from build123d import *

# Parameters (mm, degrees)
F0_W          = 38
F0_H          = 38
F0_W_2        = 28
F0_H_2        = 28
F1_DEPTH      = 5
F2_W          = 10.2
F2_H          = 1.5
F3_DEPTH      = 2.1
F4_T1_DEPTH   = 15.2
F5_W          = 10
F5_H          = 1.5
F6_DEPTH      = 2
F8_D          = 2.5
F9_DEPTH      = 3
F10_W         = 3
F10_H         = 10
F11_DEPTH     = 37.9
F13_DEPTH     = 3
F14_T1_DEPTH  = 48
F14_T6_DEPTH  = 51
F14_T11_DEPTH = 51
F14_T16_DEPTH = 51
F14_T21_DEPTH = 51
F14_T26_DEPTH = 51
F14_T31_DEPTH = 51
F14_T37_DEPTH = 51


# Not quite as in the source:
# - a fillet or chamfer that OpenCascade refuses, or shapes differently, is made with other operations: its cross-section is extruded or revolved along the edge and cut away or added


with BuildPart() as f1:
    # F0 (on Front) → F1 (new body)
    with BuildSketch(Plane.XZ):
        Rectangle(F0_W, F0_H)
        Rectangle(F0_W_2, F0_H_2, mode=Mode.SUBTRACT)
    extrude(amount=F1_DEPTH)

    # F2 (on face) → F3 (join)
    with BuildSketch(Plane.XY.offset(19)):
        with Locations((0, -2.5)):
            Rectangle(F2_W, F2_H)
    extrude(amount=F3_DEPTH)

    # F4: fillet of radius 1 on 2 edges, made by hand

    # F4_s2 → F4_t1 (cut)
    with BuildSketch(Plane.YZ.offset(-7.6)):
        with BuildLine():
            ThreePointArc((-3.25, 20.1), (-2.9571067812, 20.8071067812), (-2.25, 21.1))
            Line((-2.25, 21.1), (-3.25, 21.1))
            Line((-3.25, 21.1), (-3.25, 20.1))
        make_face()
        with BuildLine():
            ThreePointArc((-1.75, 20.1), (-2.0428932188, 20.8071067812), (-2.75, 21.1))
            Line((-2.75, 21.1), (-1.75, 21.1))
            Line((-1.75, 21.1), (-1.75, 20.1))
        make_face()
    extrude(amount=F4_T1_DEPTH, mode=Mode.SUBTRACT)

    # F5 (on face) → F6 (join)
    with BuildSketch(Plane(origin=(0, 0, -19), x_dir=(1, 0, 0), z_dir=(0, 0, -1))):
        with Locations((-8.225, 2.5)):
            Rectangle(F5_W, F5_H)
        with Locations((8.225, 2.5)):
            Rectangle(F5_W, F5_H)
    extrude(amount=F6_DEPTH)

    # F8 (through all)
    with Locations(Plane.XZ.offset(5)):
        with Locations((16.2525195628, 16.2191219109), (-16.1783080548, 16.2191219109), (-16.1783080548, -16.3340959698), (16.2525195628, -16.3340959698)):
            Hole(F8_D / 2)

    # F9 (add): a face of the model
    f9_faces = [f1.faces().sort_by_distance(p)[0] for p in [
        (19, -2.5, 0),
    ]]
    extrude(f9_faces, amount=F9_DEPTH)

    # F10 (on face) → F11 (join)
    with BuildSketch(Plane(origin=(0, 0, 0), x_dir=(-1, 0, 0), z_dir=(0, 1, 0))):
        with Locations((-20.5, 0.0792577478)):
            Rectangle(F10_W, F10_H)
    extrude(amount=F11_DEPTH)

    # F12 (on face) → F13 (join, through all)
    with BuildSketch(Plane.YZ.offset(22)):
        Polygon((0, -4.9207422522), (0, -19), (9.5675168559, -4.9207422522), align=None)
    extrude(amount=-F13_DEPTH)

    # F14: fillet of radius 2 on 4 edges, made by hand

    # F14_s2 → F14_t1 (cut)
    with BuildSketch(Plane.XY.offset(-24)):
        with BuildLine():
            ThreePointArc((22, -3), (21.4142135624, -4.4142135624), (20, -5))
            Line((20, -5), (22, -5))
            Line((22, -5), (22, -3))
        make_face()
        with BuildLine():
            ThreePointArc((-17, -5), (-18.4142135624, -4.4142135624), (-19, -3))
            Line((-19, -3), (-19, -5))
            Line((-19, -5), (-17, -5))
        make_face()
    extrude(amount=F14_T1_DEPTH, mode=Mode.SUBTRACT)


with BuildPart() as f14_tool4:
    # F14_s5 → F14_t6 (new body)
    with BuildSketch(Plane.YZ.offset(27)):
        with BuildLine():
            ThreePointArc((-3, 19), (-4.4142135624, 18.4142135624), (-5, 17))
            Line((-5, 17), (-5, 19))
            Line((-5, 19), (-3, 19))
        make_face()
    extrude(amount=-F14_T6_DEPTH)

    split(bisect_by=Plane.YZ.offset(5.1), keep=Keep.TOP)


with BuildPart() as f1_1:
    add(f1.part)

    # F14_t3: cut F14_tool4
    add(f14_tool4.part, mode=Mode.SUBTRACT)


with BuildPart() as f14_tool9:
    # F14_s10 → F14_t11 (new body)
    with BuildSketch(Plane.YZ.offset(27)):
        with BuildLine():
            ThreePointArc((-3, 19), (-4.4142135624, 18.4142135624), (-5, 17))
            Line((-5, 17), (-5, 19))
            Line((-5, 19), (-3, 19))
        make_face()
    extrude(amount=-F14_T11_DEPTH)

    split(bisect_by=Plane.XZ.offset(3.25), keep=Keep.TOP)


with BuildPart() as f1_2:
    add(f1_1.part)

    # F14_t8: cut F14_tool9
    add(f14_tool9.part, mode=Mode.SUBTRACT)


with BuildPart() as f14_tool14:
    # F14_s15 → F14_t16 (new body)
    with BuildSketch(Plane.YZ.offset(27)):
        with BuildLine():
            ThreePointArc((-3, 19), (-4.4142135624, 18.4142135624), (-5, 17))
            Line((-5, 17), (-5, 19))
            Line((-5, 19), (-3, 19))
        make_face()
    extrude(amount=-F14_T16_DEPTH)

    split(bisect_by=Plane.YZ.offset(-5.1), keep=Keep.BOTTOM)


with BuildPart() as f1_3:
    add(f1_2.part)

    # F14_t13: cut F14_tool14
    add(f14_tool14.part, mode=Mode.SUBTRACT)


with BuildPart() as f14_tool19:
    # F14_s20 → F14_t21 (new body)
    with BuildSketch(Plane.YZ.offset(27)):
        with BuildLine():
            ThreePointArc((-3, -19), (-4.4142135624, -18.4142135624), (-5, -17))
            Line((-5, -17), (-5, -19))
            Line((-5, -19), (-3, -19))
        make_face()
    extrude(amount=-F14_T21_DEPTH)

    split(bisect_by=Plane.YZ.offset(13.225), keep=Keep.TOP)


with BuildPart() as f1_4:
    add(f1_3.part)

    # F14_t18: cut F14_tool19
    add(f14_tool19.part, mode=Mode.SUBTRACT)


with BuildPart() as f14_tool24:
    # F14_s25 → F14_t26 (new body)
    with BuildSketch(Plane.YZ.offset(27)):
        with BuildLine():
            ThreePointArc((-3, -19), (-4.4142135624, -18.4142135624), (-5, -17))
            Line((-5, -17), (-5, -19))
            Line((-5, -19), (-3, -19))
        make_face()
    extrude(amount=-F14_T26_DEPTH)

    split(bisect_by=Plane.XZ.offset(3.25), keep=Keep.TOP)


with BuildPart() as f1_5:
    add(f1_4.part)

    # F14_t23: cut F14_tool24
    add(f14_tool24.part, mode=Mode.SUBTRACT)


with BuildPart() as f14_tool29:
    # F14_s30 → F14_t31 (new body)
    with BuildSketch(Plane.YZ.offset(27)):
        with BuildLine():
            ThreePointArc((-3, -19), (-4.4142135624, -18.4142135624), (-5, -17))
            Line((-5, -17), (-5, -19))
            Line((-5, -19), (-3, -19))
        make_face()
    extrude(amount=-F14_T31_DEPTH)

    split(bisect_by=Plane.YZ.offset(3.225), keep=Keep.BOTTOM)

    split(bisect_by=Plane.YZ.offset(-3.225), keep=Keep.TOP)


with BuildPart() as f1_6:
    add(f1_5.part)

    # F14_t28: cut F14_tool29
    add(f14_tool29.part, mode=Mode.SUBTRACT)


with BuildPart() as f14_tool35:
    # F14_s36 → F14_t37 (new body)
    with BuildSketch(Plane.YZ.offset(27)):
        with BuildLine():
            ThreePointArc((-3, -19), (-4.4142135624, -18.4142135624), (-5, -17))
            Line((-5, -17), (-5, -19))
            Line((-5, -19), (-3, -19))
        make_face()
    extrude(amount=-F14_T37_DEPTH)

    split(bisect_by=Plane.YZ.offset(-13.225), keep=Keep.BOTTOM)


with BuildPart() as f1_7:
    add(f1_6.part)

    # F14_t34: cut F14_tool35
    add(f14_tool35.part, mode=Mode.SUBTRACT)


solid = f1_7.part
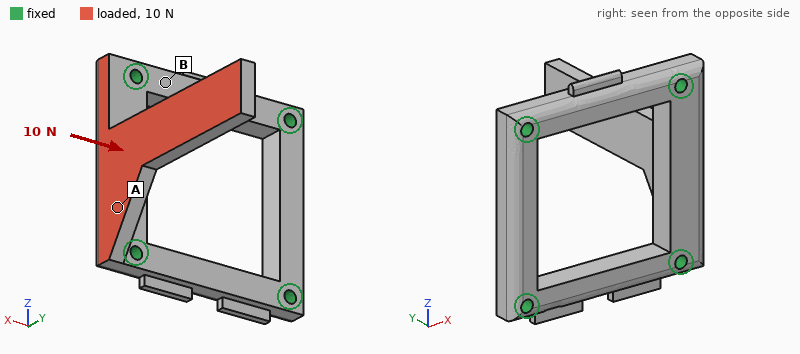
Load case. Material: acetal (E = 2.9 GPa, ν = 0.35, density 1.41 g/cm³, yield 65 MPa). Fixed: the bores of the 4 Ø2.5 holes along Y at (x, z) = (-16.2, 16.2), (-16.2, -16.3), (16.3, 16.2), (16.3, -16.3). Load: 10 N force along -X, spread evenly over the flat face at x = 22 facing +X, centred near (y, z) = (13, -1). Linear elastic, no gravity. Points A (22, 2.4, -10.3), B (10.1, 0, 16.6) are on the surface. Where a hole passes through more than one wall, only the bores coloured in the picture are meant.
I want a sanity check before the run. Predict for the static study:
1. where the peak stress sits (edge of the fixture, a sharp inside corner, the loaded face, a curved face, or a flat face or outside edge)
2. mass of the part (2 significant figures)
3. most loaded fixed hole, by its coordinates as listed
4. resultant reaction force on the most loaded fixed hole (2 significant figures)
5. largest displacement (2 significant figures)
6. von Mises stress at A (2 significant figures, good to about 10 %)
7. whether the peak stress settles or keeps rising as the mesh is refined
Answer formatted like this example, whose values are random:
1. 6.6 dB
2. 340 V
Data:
1. edge of the fixture
2. 7.1 g
3. (16.3, -16.3)
4. 6.5 N
5. 0.78 mm
6. 3.5 MPa
7. keeps rising
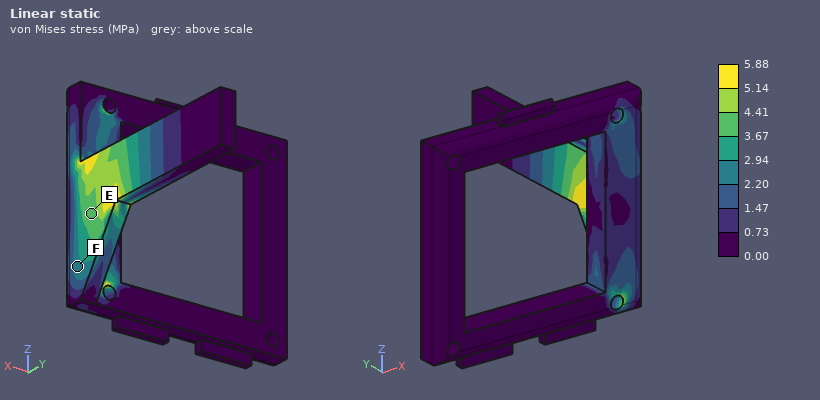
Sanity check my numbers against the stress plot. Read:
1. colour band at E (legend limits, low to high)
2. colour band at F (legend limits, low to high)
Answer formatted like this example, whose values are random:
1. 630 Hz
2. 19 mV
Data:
1. 3.67 to 4.41 MPa
2. 2.20 to 2.94 MPa
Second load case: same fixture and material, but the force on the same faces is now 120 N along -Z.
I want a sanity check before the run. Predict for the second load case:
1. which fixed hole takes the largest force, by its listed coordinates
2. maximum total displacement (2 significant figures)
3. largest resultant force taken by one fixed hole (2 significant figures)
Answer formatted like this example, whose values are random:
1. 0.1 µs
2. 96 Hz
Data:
1. (16.3, -16.3)
2. 0.77 mm
3. 100 N
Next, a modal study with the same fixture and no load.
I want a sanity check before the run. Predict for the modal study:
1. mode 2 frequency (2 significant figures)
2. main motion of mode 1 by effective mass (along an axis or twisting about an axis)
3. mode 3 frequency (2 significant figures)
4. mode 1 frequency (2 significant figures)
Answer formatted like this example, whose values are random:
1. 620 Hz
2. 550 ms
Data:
1. 1600 Hz
2. along X
3. 2500 Hz
4. 470 Hz
